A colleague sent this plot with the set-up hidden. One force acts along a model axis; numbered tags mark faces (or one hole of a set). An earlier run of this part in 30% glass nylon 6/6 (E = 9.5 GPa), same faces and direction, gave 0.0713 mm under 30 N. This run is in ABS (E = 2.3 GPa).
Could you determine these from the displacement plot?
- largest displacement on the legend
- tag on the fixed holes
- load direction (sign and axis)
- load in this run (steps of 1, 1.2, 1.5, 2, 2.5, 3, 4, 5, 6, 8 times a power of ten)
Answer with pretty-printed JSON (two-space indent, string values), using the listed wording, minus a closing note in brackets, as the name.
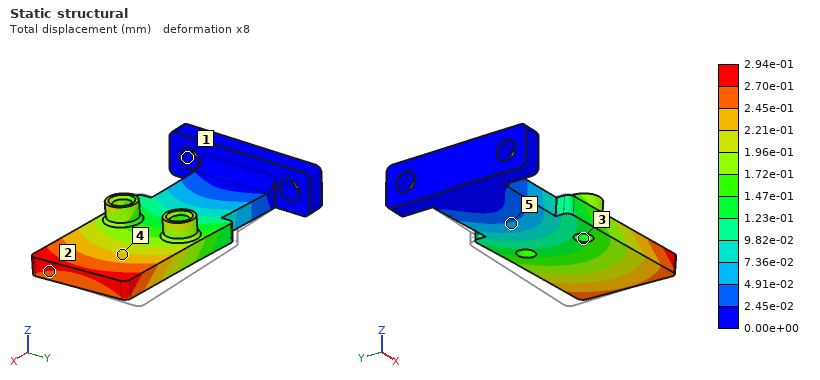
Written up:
{
  "largest displacement on the legend": "2.94e-01 mm",
  "tag on the fixed holes": "1",
  "load direction": "-Y",
  "load in this run": "30 N"
}
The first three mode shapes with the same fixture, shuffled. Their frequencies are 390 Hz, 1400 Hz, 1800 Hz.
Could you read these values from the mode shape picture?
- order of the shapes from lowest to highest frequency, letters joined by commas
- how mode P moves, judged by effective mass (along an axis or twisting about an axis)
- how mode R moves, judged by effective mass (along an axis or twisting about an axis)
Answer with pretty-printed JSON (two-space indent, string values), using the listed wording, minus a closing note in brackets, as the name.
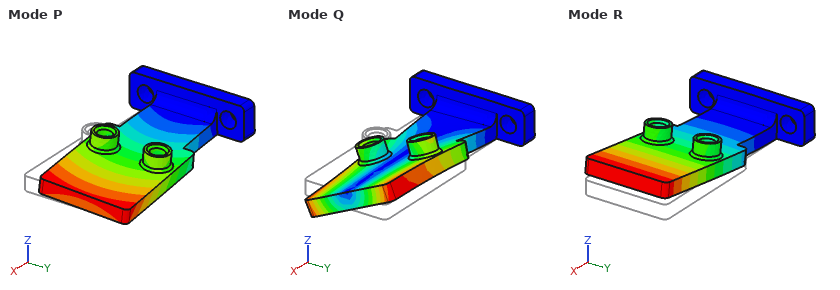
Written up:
{
  "order of the shapes from lowest to highest frequency, letters joined by commas": "R, P, Q",
  "how mode P moves, judged by effective mass": "along Y",
  "how mode R moves, judged by effective mass": "along Z"
}
